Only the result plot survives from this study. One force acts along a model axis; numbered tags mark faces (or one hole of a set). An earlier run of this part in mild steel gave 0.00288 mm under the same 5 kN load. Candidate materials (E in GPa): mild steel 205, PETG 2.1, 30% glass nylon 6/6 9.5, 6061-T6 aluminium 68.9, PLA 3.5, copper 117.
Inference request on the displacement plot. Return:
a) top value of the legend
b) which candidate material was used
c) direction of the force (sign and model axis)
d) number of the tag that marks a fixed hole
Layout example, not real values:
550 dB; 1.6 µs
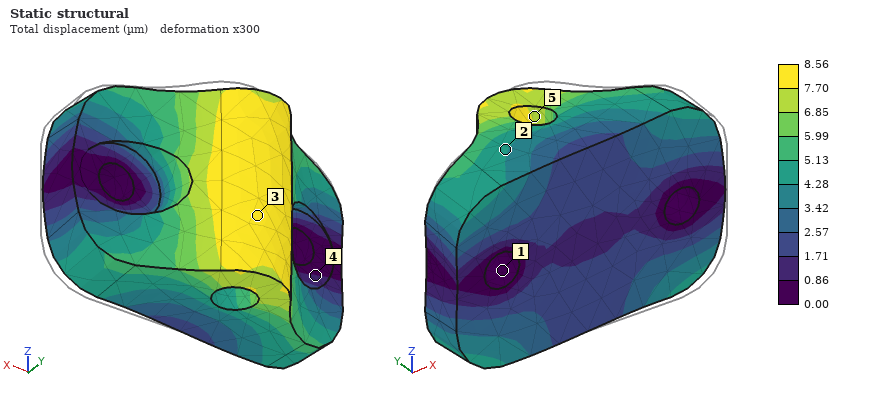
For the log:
8.56 µm; 6061-T6 aluminium; -X; 1
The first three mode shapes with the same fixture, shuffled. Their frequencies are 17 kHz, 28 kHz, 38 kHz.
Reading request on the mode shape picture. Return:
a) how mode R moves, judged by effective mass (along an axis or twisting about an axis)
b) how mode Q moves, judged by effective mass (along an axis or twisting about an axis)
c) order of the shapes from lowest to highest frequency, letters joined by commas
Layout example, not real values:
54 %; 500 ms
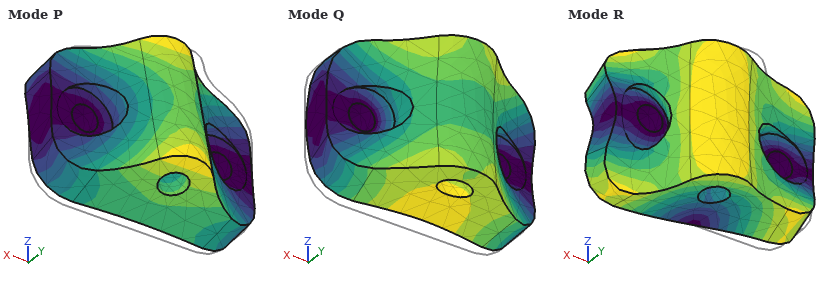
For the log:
along X; along Y; P, Q, R
